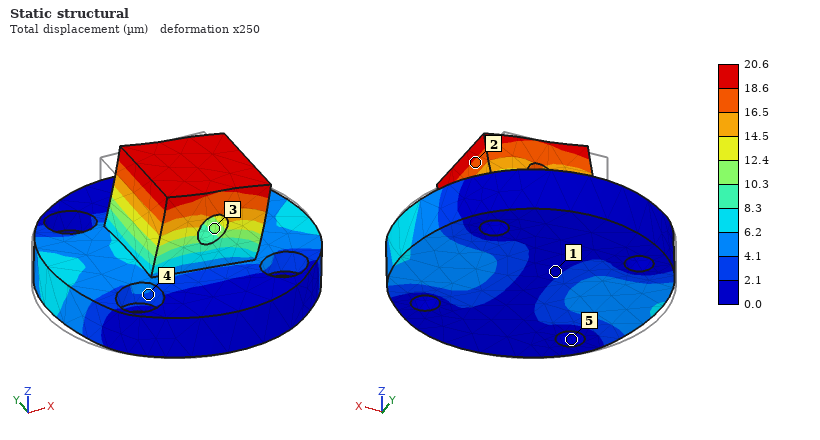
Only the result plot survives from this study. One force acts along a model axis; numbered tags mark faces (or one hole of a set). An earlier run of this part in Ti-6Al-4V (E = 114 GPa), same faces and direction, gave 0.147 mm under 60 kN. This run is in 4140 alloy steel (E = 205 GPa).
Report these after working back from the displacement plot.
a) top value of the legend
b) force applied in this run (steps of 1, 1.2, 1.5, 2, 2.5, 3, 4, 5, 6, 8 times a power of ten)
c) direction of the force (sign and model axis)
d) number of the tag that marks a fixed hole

20.6 µm
15 kN
+X
5
